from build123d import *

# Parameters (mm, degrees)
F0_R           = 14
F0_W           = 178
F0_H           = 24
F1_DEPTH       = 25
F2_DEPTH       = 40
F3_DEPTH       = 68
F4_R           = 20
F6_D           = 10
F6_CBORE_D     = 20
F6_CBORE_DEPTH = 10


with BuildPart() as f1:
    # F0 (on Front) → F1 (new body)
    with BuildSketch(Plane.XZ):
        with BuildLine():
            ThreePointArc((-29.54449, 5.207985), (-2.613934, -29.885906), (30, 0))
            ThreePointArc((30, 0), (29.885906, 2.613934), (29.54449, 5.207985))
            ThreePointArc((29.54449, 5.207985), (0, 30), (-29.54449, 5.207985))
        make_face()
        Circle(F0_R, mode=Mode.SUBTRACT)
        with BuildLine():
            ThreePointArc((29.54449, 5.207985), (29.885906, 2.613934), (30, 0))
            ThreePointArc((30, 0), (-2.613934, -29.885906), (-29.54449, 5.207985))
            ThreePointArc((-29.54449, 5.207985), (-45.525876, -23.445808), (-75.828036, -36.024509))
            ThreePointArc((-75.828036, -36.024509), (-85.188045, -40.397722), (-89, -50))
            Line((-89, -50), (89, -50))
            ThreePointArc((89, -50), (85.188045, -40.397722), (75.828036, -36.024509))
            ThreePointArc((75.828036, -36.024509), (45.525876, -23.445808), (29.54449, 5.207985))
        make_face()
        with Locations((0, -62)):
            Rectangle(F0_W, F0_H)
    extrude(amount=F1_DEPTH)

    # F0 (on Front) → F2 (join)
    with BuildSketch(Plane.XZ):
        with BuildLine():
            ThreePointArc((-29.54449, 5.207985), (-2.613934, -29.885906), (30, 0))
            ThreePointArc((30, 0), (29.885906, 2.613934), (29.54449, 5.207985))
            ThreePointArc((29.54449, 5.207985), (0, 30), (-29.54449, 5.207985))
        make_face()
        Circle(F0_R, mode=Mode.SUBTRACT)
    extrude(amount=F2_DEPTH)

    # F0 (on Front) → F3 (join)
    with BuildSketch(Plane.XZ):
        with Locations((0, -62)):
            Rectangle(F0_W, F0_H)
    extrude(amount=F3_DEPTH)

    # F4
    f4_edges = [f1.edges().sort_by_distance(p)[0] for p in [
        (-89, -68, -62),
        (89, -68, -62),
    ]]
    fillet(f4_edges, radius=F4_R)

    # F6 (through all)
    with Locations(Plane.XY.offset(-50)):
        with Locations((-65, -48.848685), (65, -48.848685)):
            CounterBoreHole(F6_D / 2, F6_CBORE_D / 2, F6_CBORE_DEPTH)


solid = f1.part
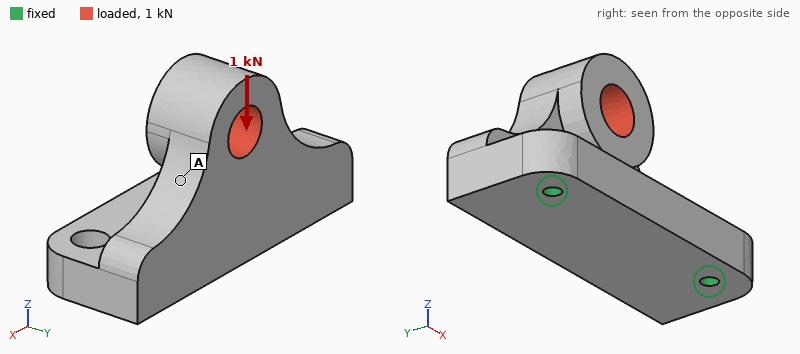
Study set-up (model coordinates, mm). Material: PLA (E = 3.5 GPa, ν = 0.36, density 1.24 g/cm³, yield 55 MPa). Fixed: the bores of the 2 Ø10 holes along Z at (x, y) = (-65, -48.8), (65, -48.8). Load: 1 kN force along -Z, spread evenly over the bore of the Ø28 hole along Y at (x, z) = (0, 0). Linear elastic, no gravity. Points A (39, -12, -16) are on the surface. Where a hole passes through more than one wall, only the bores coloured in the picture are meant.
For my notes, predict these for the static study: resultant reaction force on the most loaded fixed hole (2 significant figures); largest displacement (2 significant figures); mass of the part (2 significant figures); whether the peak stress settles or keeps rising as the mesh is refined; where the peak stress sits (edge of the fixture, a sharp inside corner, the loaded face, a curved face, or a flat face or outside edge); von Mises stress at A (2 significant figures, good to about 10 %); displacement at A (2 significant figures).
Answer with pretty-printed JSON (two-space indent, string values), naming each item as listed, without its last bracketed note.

{
  "resultant reaction force on the most loaded fixed hole": "520 N",
  "largest displacement": "0.30 mm",
  "mass of the part": "580 g",
  "whether the peak stress settles or keeps rising as the mesh is refined": "keeps rising",
  "where the peak stress sits": "edge of the fixture",
  "von Mises stress at A": "1.1 MPa",
  "displacement at A": "0.20 mm"
}
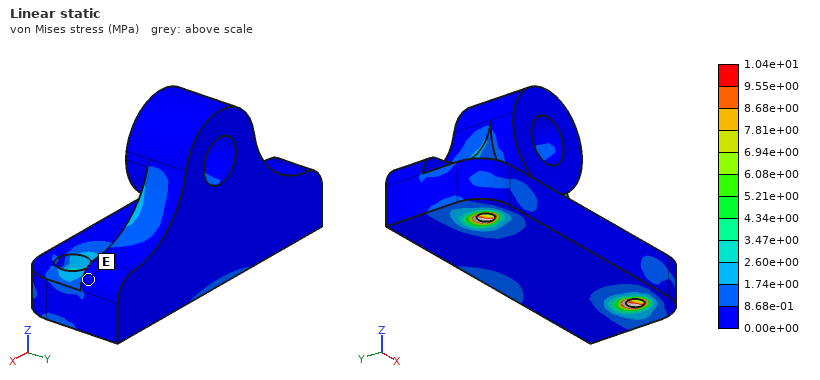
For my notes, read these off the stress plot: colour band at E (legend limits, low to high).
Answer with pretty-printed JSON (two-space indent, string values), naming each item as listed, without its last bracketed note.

{
  "colour band at E": "0.00e+00 to 8.68e-01 MPa"
}
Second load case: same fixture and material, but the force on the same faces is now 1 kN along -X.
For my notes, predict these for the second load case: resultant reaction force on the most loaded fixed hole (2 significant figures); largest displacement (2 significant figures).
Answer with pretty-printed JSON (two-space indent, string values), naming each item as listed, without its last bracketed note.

{
  "resultant reaction force on the most loaded fixed hole": "740 N",
  "largest displacement": "0.15 mm"
}
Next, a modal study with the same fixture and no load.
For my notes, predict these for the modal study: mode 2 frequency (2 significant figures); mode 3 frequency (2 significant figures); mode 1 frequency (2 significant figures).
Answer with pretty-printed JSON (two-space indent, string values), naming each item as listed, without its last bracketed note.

{
  "mode 2 frequency": "1100 Hz",
  "mode 3 frequency": "1100 Hz",
  "mode 1 frequency": "410 Hz"
}
